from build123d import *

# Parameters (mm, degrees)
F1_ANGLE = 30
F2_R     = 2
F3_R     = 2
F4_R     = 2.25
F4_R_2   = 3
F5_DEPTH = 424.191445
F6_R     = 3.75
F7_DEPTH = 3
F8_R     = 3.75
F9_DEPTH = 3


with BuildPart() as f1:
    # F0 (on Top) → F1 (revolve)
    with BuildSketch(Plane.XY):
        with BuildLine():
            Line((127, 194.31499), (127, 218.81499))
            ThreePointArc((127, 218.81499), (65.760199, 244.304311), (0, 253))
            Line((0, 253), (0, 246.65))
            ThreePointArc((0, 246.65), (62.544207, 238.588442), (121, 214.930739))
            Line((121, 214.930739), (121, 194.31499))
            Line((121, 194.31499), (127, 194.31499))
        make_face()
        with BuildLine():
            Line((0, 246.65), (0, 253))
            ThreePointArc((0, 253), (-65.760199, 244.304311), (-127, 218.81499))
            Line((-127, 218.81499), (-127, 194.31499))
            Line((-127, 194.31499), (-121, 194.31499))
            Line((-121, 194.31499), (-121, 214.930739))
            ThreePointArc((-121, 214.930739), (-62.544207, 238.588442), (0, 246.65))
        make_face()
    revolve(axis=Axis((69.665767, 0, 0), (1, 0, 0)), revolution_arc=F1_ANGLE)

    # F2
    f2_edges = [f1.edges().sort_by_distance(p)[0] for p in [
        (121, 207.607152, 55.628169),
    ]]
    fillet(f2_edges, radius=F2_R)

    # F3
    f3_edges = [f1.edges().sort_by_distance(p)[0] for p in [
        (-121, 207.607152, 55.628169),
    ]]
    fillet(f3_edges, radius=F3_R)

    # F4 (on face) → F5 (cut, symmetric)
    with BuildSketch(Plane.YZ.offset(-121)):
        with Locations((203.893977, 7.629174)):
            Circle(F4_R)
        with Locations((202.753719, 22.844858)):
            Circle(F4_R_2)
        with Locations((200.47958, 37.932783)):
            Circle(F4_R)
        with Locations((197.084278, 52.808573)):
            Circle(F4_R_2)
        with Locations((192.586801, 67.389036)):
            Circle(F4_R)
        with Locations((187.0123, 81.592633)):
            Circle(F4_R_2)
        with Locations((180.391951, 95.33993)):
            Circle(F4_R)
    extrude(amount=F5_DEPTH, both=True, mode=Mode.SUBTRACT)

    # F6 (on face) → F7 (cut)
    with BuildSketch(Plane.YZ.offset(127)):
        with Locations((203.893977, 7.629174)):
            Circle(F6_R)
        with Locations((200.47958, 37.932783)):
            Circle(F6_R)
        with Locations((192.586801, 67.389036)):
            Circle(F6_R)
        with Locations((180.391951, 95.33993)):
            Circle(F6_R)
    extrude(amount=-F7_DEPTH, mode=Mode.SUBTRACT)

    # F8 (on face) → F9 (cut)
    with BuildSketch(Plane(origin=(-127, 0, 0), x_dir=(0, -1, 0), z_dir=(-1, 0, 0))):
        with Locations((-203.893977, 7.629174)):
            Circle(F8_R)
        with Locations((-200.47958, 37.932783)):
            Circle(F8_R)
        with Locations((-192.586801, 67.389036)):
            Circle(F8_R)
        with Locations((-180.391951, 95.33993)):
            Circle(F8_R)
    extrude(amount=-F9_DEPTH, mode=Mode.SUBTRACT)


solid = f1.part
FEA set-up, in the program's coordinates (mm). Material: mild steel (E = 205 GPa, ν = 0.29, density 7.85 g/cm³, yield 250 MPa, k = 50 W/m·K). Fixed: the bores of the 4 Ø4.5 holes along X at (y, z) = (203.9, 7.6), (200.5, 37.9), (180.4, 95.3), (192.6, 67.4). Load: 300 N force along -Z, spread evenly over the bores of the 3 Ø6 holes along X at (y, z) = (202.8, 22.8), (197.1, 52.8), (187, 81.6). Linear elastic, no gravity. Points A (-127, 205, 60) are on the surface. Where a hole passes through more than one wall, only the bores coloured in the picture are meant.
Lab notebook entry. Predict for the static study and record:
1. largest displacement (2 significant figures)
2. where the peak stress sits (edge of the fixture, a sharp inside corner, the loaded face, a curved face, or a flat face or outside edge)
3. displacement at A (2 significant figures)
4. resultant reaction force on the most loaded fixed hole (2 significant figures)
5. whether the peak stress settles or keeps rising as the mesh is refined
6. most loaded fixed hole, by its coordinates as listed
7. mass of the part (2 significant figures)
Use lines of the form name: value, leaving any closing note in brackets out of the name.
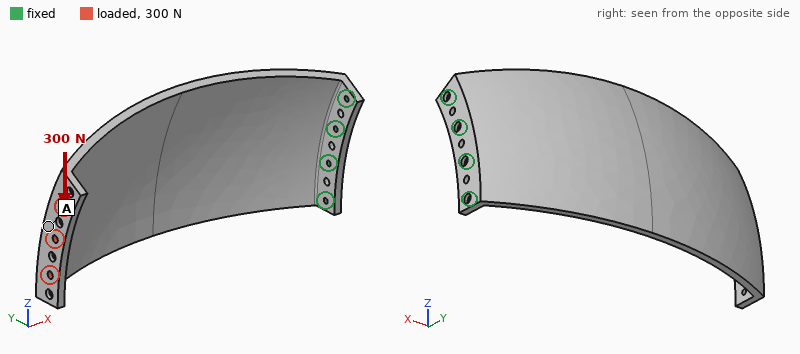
largest displacement: 1.2 mm
where the peak stress sits: edge of the fixture
displacement at A: 0.97 mm
resultant reaction force on the most loaded fixed hole: 980 N
whether the peak stress settles or keeps rising as the mesh is refined: keeps rising
most loaded fixed hole, by its coordinates as listed: (203.9, 7.6)
mass of the part: 1.8 kg
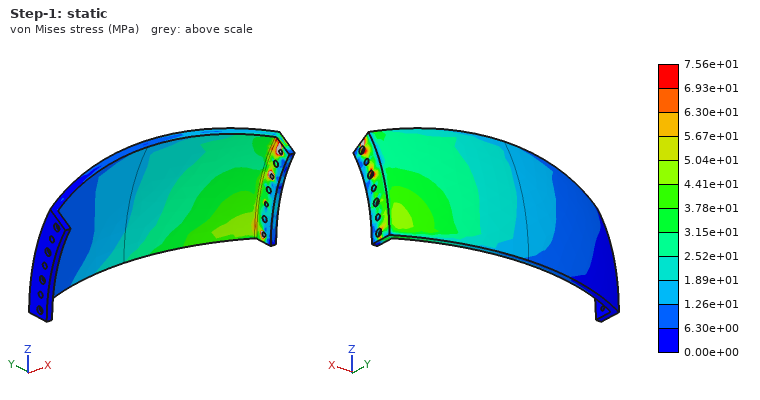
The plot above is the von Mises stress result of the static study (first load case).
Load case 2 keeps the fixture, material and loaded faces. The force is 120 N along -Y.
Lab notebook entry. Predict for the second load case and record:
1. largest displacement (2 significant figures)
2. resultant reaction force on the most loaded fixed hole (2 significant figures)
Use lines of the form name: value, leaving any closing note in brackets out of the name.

largest displacement: 1.3 mm
resultant reaction force on the most loaded fixed hole: 620 N
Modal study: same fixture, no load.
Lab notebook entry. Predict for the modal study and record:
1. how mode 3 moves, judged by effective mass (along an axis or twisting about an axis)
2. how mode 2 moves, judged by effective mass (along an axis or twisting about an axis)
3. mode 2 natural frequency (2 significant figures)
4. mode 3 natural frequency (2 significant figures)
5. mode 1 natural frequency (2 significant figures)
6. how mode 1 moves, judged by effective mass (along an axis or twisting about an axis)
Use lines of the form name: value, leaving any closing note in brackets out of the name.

how mode 3 moves, judged by effective mass: along X
how mode 2 moves, judged by effective mass: along Z
mode 2 natural frequency: 180 Hz
mode 3 natural frequency: 360 Hz
mode 1 natural frequency: 66 Hz
how mode 1 moves, judged by effective mass: along Y
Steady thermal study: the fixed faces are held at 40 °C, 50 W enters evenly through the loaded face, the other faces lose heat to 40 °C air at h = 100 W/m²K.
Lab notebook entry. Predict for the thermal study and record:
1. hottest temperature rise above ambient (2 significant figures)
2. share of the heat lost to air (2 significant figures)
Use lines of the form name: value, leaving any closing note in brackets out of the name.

hottest temperature rise above ambient: 55 K
share of the heat lost to air: 100 %
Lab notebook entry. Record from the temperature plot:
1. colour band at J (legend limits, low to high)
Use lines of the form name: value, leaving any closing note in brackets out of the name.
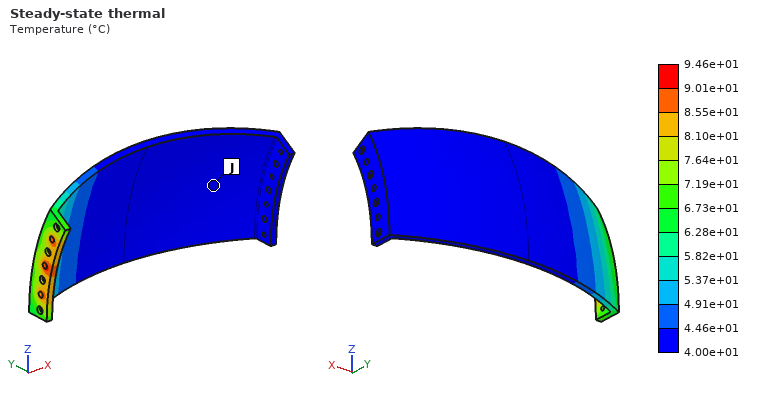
colour band at J: 4.00e+01 to 4.46e+01 °C
